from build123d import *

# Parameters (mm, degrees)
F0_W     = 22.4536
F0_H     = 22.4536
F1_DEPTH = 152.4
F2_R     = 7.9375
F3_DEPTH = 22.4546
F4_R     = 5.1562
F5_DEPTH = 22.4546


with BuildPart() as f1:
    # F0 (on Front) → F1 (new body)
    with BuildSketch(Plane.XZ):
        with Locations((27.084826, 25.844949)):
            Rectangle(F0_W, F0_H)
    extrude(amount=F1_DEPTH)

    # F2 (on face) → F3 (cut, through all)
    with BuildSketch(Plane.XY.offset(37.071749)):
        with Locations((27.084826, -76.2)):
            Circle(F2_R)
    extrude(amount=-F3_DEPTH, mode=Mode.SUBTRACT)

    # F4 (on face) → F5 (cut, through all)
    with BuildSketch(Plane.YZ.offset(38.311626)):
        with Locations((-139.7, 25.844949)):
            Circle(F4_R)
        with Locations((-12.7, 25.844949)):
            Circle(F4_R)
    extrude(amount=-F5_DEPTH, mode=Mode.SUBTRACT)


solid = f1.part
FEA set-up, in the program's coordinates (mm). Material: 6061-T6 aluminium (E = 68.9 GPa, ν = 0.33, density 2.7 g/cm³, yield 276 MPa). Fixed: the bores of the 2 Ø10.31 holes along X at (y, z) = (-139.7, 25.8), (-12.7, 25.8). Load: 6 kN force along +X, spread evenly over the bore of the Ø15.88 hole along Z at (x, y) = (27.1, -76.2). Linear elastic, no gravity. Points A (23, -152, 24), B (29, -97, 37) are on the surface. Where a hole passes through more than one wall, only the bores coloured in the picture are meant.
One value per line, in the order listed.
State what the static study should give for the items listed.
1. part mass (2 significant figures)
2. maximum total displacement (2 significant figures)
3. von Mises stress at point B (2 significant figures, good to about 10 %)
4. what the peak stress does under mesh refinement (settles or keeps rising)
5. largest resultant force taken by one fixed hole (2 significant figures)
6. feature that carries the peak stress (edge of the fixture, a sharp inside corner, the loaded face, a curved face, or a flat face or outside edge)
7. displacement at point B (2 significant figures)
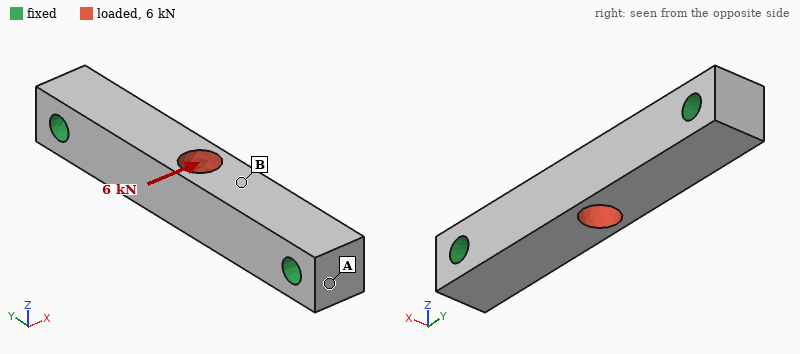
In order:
190 g
57 µm
17 MPa
keeps rising
3.0 kN
edge of the fixture
41 µm
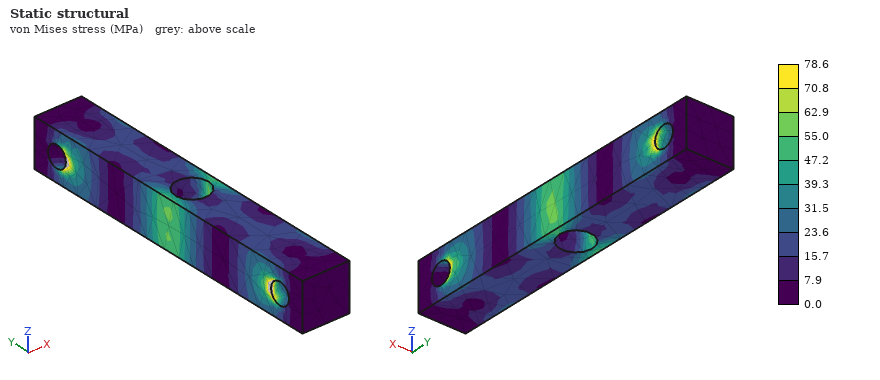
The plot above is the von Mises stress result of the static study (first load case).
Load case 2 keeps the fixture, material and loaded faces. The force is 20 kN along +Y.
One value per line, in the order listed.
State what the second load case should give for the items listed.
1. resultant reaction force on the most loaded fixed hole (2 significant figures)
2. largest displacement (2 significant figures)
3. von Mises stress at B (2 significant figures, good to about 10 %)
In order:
10 kN
18 µm
20 MPa
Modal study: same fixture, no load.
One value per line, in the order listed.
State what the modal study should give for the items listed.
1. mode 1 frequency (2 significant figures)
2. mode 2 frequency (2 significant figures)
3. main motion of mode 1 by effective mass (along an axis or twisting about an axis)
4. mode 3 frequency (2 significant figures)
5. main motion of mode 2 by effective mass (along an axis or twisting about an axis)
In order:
5700 Hz
7000 Hz
along Z
12 kHz
along X
